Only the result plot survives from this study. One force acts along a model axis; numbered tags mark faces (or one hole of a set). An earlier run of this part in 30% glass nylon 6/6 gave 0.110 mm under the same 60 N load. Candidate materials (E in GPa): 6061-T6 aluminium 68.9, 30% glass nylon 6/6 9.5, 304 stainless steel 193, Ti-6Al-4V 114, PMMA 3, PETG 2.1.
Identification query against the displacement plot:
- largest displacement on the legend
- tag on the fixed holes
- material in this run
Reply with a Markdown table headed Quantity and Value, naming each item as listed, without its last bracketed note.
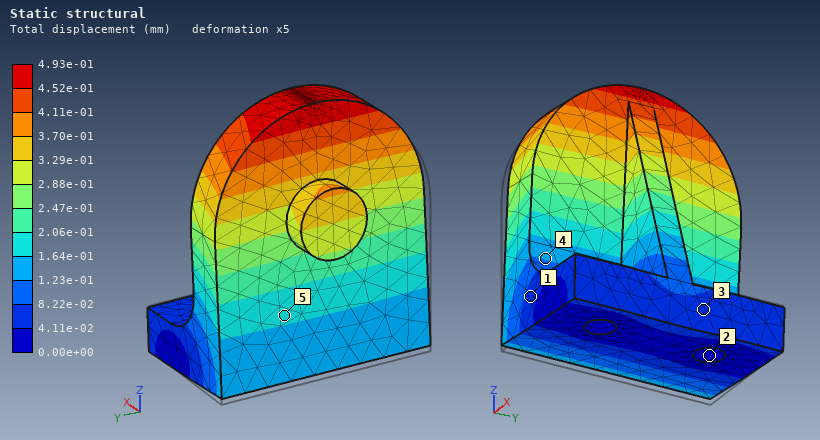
| Quantity | Value |
|---|---|
| largest displacement on the legend | 4.93e-01 mm |
| tag on the fixed holes | 2 |
| material in this run | PETG |
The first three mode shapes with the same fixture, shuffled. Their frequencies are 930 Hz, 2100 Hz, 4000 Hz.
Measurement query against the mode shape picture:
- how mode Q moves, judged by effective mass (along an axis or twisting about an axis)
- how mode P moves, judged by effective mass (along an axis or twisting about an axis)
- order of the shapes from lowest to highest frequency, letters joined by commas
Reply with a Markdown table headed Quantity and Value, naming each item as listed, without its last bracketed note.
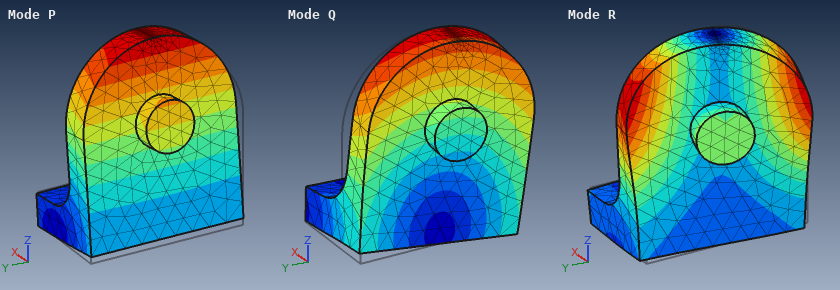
| Quantity | Value |
|---|---|
| how mode Q moves, judged by effective mass | along Y |
| how mode P moves, judged by effective mass | along X |
| order of the shapes from lowest to highest frequency, letters joined by commas | P, Q, R |
